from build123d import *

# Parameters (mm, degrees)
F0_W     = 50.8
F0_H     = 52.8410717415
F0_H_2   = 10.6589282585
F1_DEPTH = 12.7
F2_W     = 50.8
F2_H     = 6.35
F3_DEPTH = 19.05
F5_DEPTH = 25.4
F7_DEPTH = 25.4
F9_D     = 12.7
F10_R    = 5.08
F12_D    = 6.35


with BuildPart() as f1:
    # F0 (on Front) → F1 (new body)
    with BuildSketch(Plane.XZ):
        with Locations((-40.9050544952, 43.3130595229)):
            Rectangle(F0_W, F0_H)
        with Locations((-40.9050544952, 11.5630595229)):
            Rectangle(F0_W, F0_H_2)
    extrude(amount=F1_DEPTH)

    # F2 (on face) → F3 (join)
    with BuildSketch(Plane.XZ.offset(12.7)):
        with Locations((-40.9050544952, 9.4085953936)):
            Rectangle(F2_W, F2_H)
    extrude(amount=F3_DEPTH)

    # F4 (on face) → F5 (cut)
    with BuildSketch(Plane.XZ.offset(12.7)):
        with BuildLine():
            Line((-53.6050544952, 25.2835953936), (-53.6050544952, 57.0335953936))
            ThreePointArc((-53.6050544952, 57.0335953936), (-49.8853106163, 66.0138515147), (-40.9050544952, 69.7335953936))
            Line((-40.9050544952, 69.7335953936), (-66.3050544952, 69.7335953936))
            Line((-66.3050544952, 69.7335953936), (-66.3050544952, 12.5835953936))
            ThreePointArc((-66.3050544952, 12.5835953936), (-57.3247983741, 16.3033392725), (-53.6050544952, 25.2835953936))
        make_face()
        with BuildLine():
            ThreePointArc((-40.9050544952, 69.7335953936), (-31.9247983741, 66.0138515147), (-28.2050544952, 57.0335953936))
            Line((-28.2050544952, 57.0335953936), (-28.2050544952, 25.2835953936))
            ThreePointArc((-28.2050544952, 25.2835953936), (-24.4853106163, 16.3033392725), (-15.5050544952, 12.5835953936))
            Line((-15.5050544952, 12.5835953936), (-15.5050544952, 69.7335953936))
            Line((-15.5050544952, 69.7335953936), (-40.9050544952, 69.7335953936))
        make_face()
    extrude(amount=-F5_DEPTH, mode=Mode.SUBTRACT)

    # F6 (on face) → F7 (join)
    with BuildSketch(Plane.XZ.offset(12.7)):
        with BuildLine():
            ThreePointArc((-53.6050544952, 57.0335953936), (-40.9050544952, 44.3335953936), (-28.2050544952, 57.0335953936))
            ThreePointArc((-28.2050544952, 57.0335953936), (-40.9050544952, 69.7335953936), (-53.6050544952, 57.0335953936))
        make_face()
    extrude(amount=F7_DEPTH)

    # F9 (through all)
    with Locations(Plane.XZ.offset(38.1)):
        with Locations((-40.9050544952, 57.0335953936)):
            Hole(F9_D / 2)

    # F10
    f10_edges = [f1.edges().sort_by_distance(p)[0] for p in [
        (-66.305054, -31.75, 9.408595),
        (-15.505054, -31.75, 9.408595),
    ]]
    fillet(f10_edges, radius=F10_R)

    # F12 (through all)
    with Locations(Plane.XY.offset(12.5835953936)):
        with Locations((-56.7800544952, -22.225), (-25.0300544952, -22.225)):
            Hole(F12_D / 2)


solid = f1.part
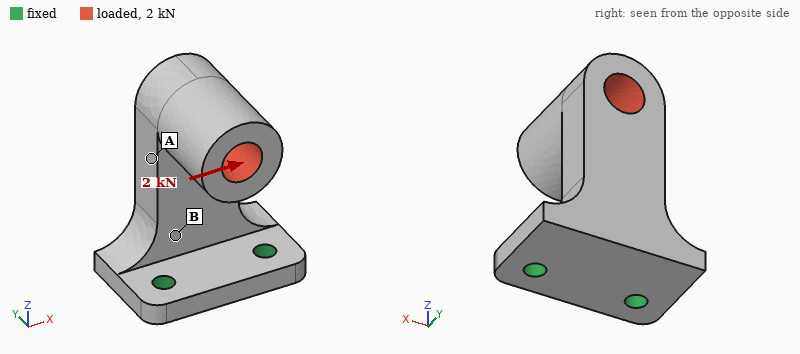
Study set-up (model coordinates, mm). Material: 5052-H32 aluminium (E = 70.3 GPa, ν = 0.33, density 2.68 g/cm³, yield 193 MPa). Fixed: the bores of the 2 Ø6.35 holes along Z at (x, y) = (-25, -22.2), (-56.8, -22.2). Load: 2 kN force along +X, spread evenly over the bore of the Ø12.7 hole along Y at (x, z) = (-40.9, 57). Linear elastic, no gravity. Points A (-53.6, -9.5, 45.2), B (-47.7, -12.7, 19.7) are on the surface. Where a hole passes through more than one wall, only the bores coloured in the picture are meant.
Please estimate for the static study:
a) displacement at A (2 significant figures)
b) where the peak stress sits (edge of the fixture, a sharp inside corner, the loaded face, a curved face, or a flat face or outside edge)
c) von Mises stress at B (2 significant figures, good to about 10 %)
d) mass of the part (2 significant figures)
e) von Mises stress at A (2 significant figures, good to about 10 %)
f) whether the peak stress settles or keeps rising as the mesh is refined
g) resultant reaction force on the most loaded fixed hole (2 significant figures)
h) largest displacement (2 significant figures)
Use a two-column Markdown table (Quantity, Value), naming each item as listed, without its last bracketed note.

| Quantity | Value |
|---|---|
| displacement at A | 0.14 mm |
| where the peak stress sits | edge of the fixture |
| von Mises stress at B | 64 MPa |
| mass of the part | 97 g |
| von Mises stress at A | 34 MPa |
| whether the peak stress settles or keeps rising as the mesh is refined | keeps rising |
| resultant reaction force on the most loaded fixed hole | 3.0 kN |
| largest displacement | 0.34 mm |
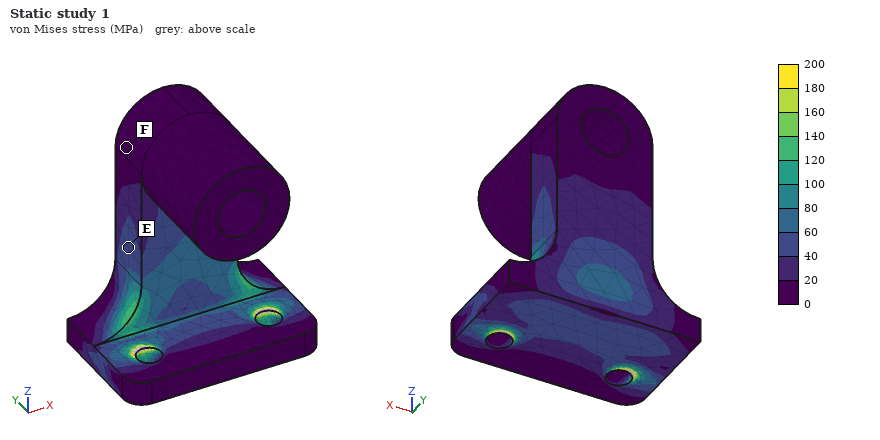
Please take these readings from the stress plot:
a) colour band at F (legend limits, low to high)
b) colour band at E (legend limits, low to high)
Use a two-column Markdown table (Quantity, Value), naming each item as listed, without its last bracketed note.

| Quantity | Value |
|---|---|
| colour band at F | 0 to 20 MPa |
| colour band at E | 40 to 60 MPa |
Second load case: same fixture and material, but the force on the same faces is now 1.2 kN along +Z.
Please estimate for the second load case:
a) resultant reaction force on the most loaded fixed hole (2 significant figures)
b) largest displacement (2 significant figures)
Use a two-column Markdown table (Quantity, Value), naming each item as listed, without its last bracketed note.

| Quantity | Value |
|---|---|
| resultant reaction force on the most loaded fixed hole | 610 N |
| largest displacement | 0.14 mm |
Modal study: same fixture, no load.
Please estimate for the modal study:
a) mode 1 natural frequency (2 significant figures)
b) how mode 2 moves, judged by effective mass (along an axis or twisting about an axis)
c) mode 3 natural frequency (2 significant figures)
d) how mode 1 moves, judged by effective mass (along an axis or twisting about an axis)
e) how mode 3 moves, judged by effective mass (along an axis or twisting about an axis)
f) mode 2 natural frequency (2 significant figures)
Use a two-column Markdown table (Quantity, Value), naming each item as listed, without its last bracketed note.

| Quantity | Value |
|---|---|
| mode 1 natural frequency | 1000 Hz |
| how mode 2 moves, judged by effective mass | along X |
| mode 3 natural frequency | 4500 Hz |
| how mode 1 moves, judged by effective mass | along Y |
| how mode 3 moves, judged by effective mass | along Z |
| mode 2 natural frequency | 2300 Hz |
